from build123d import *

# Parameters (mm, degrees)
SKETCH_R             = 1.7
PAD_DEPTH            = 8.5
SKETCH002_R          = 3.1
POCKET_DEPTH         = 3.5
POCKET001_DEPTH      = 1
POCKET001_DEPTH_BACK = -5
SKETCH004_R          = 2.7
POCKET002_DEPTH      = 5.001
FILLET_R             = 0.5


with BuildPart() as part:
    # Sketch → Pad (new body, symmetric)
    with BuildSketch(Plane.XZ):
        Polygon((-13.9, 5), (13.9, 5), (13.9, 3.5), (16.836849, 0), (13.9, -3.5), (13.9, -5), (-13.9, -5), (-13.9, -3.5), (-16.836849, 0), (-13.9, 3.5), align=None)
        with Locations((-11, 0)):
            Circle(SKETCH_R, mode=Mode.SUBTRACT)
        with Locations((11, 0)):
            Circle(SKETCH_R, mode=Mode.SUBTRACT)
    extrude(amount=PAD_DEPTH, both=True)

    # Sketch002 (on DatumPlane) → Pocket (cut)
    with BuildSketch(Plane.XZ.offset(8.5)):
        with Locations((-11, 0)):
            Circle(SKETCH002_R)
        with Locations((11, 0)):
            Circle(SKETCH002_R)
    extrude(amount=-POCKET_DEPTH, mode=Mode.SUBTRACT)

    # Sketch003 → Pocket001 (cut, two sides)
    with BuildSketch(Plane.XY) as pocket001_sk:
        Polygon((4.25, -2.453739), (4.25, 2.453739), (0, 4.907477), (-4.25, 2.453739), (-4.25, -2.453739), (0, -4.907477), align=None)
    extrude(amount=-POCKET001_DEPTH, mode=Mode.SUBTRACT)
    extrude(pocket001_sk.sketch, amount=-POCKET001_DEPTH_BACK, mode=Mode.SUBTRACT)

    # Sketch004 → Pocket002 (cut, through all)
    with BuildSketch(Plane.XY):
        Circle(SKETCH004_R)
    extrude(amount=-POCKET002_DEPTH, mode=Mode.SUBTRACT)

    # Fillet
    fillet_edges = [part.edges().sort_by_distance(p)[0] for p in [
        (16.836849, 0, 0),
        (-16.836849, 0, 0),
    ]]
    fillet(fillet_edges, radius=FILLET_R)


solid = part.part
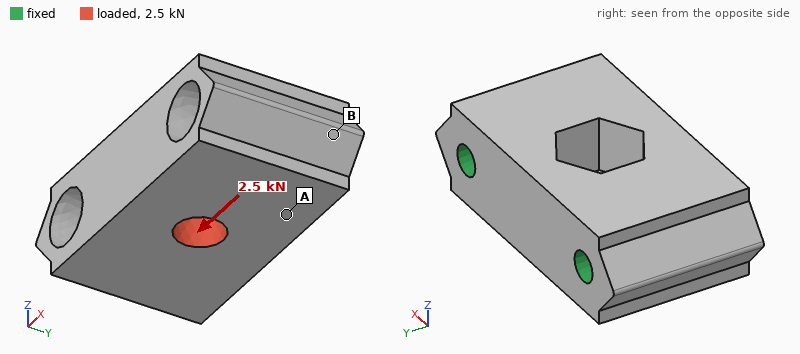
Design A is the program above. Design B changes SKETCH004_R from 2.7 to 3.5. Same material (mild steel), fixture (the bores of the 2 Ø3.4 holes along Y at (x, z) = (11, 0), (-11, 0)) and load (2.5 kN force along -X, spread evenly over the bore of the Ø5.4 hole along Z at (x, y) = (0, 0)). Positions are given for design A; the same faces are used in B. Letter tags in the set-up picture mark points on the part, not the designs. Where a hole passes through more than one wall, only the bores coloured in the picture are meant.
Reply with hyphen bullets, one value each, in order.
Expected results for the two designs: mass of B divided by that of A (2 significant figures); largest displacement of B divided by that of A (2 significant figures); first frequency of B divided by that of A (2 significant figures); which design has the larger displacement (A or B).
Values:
- 0.98
- 0.89
- 1.0
- A
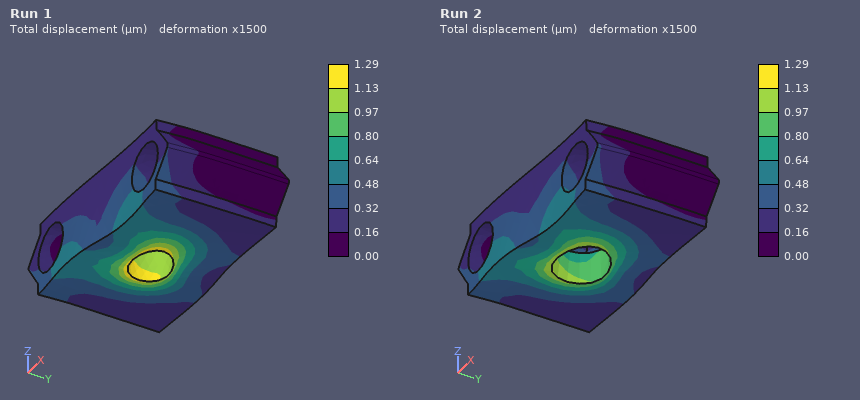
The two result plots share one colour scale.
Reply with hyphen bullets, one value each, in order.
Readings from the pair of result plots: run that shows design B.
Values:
- Run 2
